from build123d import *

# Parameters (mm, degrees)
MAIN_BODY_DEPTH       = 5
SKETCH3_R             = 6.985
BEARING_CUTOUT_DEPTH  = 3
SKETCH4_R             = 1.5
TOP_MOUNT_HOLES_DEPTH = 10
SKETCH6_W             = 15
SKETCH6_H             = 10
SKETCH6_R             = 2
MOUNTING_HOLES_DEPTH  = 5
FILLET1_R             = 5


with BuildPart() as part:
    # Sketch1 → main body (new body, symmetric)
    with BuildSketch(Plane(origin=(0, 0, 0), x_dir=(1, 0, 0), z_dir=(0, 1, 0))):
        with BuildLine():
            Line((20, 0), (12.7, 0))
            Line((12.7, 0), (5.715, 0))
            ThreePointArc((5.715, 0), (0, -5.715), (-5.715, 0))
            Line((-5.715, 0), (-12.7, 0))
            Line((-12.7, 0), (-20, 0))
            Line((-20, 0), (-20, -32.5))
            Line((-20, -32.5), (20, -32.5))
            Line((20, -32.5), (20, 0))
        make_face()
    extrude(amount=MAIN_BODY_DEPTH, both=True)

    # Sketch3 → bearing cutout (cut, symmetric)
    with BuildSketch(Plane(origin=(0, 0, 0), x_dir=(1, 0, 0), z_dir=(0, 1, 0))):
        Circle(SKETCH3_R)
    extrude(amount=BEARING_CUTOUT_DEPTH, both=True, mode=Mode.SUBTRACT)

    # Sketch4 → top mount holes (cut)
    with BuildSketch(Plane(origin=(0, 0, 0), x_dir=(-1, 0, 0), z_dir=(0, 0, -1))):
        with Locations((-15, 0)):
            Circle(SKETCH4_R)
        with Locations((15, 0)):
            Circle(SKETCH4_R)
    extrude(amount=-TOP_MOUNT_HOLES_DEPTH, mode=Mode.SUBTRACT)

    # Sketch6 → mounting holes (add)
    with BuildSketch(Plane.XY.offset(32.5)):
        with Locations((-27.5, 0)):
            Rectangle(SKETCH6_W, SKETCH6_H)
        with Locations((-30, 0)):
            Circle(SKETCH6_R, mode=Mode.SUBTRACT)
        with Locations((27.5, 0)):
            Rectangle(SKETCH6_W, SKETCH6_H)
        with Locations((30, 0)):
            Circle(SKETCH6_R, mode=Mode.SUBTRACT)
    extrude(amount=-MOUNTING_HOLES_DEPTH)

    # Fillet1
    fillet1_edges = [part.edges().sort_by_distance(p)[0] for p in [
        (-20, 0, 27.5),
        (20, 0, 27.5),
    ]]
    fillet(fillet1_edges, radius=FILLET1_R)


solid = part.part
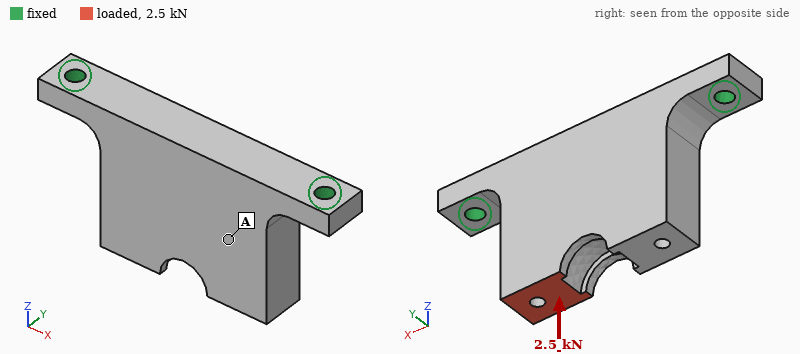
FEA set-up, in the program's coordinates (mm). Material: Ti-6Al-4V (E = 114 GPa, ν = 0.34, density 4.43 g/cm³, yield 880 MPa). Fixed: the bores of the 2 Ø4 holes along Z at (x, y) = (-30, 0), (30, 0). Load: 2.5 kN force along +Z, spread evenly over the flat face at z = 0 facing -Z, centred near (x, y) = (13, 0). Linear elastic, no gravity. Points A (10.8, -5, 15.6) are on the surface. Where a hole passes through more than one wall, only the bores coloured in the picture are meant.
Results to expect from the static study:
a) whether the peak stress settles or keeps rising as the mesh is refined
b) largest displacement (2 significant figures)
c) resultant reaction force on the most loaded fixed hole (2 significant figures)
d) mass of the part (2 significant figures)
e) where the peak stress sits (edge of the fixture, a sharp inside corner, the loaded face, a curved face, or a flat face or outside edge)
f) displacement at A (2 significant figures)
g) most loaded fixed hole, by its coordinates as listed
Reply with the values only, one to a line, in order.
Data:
keeps rising
29 µm
2.1 kN
61 g
edge of the fixture
21 µm
(30, 0)
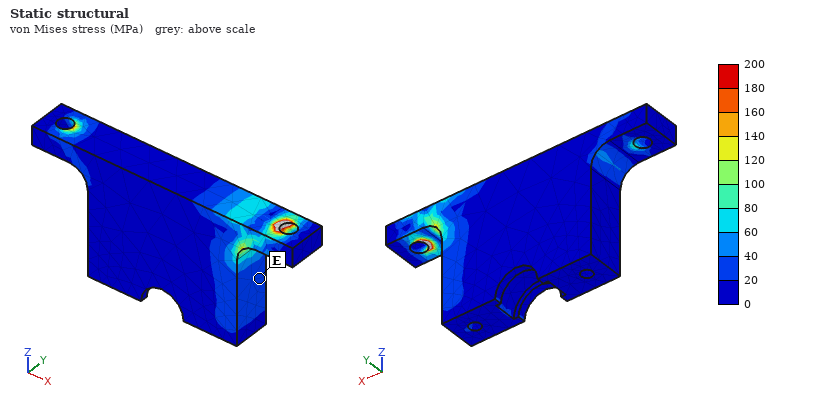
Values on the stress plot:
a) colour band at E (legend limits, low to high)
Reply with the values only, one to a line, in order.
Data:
20 to 40 MPa
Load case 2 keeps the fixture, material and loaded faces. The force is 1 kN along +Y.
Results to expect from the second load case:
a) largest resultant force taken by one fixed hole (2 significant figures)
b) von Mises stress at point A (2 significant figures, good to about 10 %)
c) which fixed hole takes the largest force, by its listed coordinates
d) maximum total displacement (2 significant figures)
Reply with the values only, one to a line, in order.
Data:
760 N
44 MPa
(30, 0)
0.34 mm
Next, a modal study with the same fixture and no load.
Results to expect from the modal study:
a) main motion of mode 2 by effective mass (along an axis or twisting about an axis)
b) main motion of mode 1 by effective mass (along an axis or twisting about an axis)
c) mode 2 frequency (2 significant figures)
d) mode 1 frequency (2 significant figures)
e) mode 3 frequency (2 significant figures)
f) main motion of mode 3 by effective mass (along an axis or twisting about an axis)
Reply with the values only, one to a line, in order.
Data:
along Z
along Y
8400 Hz
2300 Hz
10 kHz
twisting about Z
